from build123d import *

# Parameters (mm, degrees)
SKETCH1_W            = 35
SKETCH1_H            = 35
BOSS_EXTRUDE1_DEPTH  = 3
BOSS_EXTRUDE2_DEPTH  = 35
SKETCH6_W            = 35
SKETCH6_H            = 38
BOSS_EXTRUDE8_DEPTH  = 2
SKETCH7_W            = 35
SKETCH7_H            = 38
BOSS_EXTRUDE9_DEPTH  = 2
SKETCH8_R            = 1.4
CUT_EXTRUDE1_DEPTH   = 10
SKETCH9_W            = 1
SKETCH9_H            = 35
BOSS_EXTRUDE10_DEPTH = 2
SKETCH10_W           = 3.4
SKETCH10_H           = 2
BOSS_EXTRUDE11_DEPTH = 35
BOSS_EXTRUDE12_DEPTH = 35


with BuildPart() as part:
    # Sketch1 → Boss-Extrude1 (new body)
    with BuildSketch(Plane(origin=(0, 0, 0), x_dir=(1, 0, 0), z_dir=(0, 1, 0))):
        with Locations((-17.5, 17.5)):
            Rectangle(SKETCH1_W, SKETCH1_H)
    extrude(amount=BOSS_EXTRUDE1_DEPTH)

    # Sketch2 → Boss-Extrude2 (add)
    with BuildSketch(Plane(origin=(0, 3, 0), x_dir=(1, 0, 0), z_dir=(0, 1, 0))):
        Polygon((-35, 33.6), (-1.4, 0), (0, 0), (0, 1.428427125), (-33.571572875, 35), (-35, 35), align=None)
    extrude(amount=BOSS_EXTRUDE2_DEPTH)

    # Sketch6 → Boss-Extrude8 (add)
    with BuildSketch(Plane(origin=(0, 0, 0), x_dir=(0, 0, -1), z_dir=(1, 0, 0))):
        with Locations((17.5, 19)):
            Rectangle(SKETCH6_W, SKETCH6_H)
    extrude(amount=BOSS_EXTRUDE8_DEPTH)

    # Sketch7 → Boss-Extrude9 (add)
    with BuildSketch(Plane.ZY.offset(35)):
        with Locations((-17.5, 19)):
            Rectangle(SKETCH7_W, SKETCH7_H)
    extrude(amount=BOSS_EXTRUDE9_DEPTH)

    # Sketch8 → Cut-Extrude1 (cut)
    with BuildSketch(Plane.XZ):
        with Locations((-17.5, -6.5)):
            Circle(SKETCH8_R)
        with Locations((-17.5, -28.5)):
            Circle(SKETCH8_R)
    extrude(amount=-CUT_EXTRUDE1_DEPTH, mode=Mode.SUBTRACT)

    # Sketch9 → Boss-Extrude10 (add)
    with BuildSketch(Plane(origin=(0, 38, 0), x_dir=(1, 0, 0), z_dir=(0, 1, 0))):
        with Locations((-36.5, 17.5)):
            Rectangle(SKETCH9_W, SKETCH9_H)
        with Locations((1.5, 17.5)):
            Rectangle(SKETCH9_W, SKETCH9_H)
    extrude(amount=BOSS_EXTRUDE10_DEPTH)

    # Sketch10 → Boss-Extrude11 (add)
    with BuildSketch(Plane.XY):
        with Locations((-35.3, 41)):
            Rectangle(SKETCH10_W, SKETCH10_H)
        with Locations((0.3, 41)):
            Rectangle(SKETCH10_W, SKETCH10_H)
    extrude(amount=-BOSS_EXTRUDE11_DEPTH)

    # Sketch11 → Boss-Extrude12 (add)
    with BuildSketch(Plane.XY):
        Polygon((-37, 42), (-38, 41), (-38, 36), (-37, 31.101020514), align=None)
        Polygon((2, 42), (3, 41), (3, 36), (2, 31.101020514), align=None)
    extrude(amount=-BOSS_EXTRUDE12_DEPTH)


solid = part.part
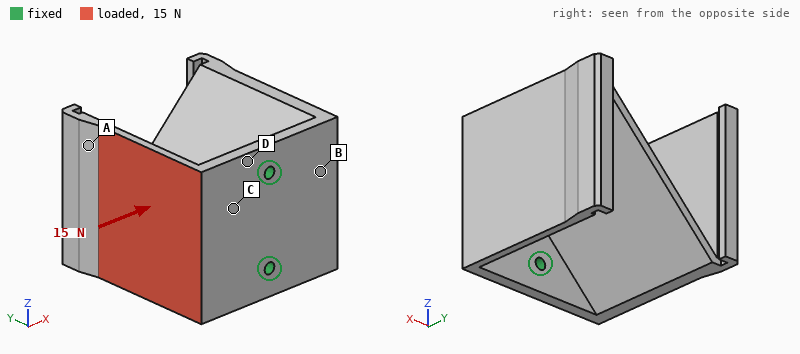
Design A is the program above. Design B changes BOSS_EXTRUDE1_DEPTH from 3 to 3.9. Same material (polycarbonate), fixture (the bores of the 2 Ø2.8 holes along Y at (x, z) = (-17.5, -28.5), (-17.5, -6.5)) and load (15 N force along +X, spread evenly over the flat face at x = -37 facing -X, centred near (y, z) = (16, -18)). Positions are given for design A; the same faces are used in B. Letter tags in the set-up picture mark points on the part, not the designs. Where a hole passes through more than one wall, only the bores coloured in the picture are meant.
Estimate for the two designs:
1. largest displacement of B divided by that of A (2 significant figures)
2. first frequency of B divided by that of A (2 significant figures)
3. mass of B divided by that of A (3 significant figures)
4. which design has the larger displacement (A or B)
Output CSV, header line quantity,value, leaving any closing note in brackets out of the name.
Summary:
quantity,value
largest displacement of B divided by that of A,0.74
first frequency of B divided by that of A,1.2
mass of B divided by that of A,1.07
which design has the larger displacement,A
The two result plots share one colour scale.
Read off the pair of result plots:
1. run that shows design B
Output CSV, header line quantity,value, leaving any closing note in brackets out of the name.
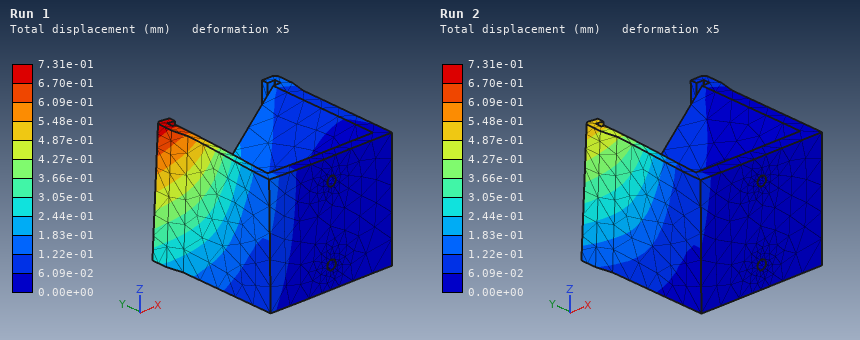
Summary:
quantity,value
run that shows design B,Run 2
